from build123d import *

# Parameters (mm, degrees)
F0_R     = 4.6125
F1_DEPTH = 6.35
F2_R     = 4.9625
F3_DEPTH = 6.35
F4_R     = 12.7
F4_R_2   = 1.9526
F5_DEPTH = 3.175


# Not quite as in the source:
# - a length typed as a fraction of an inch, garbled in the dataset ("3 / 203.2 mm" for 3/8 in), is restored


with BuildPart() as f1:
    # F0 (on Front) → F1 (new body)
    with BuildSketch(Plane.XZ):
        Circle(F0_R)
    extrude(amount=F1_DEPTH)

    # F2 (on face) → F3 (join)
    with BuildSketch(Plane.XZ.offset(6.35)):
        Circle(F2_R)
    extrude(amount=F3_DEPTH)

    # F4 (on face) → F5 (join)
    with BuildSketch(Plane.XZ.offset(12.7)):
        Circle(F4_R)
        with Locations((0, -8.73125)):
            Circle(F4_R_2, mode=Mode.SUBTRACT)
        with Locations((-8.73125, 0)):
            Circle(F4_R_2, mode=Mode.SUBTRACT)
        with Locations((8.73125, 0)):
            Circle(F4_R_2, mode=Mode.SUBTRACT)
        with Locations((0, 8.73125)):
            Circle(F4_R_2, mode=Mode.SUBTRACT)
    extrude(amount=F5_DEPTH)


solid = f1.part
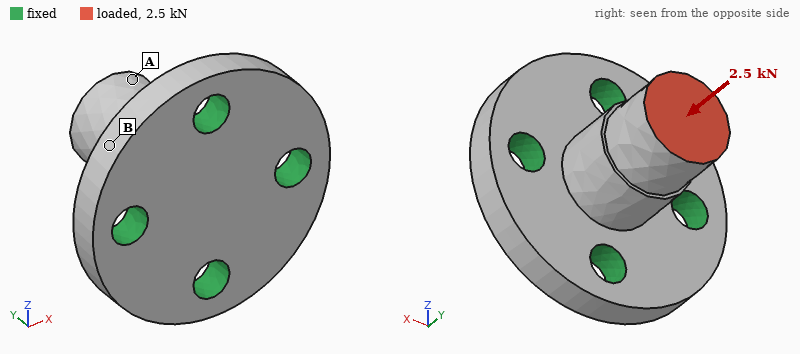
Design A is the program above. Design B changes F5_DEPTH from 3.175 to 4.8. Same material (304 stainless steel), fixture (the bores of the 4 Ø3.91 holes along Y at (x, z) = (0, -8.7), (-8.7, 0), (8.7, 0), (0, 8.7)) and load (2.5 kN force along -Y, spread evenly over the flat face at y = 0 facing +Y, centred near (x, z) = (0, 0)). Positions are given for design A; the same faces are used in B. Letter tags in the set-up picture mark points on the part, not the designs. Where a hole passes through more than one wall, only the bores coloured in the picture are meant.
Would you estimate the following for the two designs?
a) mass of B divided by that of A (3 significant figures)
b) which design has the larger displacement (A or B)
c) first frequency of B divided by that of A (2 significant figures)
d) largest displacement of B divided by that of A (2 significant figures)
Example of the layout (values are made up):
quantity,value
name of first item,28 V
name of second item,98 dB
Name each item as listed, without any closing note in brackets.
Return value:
quantity,value
mass of B divided by that of A,1.31
which design has the larger displacement,A
first frequency of B divided by that of A,1.1
largest displacement of B divided by that of A,0.80
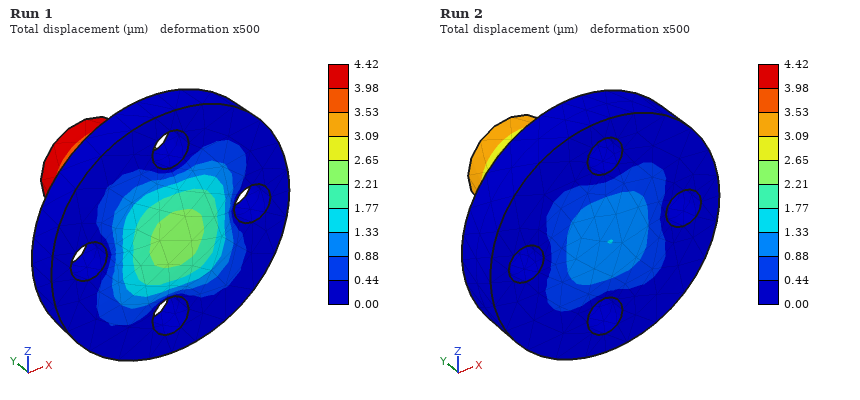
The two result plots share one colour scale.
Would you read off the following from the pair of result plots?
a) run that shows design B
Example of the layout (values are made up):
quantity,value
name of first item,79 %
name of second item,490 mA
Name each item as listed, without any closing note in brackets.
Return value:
quantity,value
run that shows design B,Run 2
